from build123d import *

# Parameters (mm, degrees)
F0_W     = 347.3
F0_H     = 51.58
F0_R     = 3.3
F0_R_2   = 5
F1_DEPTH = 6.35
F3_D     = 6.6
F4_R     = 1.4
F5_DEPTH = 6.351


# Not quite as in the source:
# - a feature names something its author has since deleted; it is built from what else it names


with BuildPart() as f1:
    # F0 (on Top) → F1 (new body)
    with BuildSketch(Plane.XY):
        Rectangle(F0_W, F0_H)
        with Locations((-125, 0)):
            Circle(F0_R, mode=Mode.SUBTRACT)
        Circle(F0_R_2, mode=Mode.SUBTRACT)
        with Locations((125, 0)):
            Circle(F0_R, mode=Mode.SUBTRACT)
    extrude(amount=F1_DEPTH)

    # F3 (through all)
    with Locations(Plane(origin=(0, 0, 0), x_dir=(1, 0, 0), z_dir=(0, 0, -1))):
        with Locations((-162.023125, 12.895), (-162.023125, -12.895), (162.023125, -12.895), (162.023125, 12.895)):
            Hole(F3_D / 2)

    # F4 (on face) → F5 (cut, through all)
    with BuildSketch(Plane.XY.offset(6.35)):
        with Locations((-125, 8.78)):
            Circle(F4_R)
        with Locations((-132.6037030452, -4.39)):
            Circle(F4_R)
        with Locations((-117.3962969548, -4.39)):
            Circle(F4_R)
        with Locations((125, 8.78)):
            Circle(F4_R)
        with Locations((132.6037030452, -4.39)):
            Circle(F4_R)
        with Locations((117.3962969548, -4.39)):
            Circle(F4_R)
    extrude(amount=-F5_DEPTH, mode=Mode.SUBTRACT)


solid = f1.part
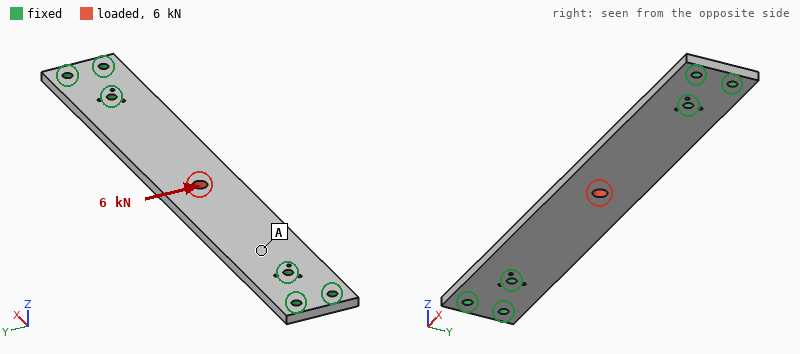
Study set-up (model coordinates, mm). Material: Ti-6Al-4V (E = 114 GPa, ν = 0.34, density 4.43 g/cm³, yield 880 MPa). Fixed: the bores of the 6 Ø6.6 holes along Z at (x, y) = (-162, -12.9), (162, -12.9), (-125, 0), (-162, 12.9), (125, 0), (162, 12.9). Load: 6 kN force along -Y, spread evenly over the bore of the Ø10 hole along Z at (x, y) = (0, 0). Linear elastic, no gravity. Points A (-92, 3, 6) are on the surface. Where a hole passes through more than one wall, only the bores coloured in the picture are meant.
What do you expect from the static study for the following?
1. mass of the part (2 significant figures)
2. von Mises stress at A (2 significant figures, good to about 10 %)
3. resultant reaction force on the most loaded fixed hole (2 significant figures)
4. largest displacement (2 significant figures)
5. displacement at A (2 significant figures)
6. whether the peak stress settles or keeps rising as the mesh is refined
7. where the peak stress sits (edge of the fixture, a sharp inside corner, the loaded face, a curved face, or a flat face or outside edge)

490 g
23 MPa
5.3 kN
0.12 mm
0.033 mm
keeps rising
edge of the fixture
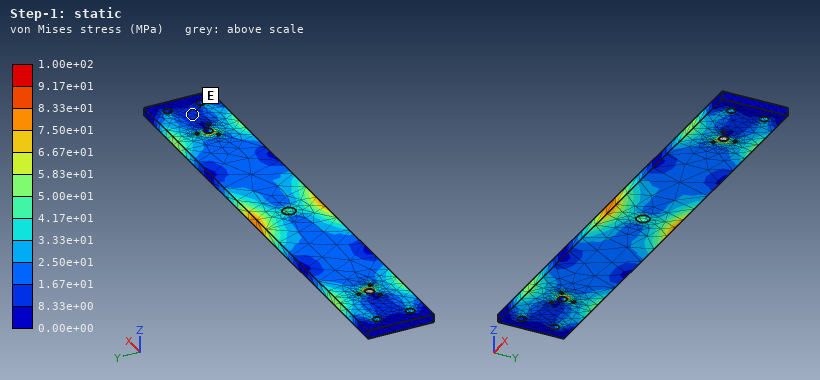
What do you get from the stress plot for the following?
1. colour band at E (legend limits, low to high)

8.33e+00 to 1.67e+01 MPa
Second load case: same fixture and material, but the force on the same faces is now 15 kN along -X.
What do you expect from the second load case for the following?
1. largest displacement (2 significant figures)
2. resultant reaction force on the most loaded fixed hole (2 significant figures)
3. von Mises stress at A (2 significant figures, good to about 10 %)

33 µm
5.1 kN
25 MPa
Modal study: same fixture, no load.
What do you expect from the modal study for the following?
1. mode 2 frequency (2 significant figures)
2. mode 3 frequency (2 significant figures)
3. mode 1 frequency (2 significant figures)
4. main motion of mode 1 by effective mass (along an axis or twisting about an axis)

1400 Hz
1500 Hz
520 Hz
along Z
